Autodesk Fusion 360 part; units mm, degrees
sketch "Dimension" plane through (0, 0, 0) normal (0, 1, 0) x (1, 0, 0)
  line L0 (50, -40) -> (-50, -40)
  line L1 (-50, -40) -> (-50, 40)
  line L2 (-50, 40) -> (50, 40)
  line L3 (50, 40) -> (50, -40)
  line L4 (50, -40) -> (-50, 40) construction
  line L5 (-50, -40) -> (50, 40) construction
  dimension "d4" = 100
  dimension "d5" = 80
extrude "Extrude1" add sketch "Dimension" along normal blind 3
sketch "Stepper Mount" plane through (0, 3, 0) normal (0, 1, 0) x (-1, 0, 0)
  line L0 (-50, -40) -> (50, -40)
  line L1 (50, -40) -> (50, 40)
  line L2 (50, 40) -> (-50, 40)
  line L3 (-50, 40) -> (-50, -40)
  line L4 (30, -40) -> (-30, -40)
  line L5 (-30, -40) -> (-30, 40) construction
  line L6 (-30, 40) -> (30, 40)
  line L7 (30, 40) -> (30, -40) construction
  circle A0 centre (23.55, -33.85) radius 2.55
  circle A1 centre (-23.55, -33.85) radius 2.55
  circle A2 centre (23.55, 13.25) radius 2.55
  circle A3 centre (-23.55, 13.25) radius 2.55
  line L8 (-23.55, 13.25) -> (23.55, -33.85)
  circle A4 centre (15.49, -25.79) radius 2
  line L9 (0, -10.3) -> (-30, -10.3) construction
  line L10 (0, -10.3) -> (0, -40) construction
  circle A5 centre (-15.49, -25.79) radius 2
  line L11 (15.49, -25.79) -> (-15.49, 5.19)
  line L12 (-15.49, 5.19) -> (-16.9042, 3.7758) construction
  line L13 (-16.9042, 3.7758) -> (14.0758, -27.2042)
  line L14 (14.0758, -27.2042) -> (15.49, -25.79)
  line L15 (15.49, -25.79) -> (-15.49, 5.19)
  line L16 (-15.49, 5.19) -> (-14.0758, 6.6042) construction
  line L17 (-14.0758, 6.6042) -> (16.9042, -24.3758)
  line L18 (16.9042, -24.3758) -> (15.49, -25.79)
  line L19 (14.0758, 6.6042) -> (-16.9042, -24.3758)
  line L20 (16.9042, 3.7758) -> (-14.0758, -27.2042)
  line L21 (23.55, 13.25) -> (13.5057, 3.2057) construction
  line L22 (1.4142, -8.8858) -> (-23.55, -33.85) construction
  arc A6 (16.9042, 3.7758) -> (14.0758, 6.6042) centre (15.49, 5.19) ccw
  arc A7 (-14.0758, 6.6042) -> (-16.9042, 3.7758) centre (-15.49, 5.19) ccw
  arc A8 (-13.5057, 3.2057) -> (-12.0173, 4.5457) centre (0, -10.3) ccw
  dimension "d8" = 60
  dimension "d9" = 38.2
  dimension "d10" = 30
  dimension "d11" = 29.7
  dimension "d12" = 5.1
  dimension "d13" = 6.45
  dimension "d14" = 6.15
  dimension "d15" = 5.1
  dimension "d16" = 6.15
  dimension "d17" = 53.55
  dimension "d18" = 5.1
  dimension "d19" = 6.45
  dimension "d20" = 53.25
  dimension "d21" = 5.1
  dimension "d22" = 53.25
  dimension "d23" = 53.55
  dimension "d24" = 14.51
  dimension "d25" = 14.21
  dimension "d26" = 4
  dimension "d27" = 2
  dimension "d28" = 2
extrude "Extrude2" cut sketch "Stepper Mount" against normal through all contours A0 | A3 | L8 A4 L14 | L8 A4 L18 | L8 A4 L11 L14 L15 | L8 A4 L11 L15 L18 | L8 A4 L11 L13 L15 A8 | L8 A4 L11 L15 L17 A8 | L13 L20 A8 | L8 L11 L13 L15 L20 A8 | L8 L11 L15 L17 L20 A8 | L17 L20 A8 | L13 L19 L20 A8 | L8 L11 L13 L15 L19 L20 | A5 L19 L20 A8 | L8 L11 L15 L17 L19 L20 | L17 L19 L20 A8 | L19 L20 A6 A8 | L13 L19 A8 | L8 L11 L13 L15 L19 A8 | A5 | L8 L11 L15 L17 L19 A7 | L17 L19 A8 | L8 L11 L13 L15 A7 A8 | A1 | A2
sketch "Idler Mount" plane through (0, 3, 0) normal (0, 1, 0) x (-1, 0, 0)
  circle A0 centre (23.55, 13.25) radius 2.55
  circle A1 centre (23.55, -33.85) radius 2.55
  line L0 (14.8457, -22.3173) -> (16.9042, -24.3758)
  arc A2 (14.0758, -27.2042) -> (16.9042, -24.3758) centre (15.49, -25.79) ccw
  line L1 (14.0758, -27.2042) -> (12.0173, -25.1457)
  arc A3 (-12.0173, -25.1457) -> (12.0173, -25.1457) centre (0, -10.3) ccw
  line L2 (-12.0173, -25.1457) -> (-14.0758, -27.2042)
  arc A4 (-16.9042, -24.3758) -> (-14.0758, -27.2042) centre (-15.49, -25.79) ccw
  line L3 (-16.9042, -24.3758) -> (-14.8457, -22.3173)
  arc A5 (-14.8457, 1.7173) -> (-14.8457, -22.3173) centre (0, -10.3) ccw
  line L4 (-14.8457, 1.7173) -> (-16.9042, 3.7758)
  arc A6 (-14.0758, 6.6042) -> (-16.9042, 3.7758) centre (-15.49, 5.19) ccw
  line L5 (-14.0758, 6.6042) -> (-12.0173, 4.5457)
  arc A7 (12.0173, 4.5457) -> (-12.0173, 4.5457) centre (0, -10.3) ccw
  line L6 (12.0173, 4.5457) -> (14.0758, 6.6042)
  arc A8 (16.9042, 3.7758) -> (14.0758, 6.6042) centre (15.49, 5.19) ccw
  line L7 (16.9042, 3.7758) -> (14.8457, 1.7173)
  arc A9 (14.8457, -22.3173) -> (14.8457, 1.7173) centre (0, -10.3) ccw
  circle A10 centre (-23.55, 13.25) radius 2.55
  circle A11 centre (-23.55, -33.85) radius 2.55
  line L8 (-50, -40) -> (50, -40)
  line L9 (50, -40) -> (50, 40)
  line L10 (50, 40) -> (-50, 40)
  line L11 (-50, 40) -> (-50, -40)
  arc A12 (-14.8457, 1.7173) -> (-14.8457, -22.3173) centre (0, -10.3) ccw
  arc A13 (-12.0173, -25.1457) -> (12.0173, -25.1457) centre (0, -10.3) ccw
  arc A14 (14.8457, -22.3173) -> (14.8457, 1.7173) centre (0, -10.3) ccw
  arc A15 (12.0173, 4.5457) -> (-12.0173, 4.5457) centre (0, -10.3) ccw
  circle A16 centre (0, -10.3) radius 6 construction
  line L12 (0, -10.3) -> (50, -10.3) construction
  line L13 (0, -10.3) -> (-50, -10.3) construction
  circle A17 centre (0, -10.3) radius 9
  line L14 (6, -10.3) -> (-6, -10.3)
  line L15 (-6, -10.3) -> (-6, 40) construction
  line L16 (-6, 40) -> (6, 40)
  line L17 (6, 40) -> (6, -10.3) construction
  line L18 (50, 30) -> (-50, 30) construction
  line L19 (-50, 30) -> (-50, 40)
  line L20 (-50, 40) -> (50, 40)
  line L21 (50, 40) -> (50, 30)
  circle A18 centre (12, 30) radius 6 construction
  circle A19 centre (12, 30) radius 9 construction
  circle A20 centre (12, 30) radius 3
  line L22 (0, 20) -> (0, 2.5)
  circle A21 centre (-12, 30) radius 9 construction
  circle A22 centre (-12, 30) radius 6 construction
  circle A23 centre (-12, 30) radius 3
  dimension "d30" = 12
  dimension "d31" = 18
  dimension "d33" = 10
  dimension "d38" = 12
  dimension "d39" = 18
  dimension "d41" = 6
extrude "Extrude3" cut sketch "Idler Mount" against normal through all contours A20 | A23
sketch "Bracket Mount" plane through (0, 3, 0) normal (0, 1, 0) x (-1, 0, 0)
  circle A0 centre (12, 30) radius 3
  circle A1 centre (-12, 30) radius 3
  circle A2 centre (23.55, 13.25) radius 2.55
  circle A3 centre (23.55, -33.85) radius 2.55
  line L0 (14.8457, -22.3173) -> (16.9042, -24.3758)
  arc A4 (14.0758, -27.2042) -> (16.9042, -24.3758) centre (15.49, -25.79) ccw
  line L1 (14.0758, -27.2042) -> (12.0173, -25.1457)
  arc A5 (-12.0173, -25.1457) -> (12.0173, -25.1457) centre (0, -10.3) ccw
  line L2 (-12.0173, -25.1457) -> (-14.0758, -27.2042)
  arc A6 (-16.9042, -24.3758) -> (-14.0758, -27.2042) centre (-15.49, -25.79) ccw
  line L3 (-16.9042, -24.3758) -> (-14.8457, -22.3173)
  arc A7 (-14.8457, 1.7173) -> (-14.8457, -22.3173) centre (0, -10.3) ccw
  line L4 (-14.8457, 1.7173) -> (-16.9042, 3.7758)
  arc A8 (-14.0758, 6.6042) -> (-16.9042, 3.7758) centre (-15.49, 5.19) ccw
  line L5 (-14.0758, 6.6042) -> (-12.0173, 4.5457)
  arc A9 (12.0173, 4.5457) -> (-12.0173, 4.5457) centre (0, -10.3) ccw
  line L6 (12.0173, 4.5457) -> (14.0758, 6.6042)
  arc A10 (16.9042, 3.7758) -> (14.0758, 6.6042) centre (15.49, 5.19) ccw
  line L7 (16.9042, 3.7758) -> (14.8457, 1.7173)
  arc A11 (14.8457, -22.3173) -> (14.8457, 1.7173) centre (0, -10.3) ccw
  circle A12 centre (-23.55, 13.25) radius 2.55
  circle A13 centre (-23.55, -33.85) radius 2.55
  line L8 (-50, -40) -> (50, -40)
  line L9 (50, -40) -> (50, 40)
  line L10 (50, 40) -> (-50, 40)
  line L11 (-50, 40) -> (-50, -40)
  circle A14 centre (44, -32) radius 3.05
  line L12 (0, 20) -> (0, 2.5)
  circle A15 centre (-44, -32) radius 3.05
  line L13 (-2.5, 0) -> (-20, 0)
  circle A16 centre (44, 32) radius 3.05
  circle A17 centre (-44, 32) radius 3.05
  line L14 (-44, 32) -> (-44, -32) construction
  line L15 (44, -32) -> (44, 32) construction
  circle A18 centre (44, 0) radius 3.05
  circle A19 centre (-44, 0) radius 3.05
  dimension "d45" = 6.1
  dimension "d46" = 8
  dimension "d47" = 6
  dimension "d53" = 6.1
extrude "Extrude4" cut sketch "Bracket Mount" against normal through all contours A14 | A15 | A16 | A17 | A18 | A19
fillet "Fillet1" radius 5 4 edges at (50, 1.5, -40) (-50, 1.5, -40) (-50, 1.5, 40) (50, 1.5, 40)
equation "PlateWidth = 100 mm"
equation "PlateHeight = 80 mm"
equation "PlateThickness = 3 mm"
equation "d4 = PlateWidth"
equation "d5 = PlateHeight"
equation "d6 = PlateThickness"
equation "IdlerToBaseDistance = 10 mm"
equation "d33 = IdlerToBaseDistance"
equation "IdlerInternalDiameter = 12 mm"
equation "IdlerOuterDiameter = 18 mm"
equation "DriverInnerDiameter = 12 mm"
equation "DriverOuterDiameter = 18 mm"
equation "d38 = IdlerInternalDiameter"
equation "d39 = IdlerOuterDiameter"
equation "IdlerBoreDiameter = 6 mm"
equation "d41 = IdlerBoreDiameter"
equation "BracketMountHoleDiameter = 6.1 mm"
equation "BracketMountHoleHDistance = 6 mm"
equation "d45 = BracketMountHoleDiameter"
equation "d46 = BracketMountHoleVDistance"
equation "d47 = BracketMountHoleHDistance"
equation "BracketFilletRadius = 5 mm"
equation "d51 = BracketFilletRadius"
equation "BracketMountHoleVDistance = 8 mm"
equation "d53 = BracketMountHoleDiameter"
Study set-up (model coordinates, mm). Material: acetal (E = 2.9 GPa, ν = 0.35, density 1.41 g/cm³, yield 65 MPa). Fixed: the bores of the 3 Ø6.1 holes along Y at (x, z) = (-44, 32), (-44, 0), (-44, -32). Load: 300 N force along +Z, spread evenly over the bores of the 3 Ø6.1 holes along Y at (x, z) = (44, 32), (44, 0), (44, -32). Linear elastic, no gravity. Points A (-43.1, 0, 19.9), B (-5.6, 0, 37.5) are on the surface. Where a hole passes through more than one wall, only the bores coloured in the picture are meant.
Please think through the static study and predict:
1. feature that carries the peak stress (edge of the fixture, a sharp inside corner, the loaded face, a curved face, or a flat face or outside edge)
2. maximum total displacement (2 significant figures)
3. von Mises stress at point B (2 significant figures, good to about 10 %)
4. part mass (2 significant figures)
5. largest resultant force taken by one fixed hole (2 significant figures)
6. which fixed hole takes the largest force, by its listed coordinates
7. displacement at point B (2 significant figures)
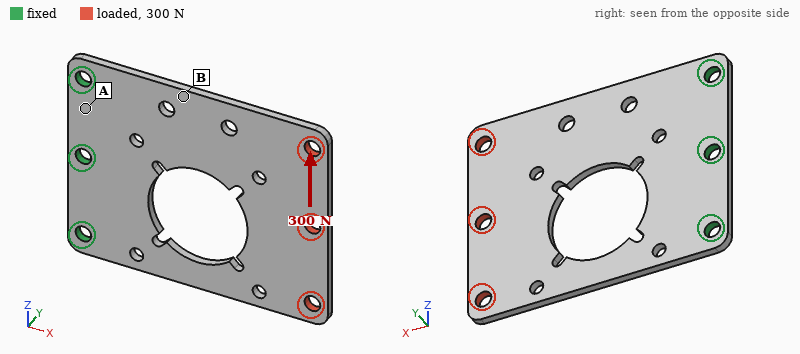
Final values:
a curved face
0.77 mm
8.2 MPa
27 g
460 N
(-44, 32)
0.27 mm
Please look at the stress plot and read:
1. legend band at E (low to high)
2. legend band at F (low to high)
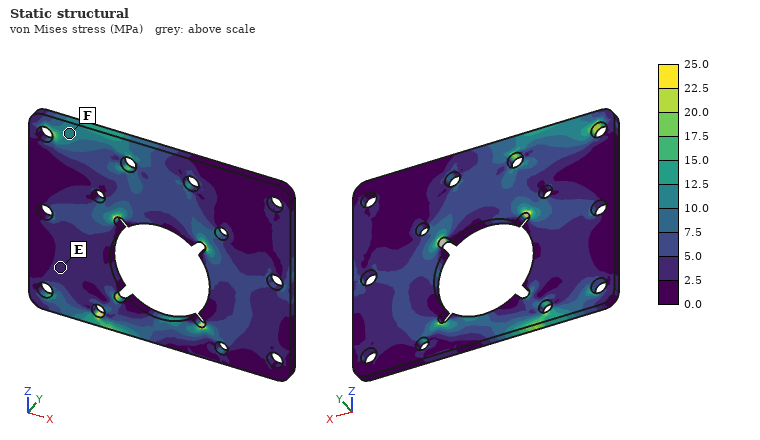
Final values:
2.5 to 5.0 MPa
10.0 to 12.5 MPa
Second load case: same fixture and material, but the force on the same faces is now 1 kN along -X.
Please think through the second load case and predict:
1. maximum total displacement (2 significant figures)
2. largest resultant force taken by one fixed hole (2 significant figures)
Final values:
0.37 mm
390 N
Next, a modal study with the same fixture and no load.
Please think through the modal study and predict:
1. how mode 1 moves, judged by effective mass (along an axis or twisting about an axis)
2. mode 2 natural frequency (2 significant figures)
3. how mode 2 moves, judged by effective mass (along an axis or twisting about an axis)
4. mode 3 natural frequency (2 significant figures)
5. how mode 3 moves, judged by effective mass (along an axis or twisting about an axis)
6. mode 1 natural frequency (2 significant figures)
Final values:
along Y
200 Hz
twisting about X
490 Hz
along Y
72 Hz
